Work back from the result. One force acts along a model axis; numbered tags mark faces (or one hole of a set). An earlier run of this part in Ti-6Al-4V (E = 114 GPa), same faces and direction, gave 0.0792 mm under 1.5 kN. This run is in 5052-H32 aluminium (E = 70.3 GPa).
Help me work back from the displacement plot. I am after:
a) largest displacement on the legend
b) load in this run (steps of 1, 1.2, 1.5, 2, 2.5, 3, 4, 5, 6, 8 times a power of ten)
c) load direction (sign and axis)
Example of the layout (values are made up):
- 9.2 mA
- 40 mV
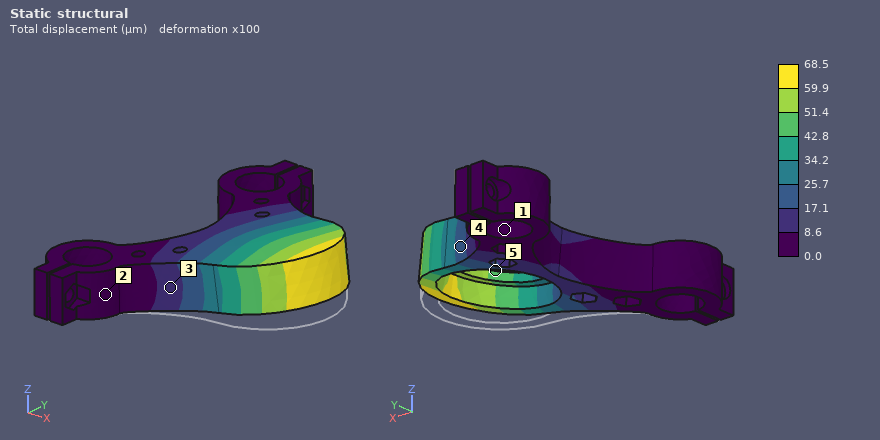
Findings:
- 68.5 µm
- 800 N
- +Z
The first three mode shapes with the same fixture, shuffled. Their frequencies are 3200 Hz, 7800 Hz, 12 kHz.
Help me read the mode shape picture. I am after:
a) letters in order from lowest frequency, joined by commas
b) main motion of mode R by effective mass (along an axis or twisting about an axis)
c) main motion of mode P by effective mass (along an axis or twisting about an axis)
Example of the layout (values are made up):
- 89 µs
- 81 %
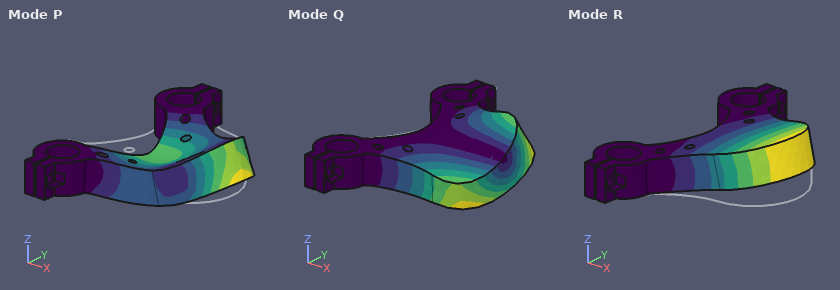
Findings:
- R, Q, P
- along Z
- along Z
